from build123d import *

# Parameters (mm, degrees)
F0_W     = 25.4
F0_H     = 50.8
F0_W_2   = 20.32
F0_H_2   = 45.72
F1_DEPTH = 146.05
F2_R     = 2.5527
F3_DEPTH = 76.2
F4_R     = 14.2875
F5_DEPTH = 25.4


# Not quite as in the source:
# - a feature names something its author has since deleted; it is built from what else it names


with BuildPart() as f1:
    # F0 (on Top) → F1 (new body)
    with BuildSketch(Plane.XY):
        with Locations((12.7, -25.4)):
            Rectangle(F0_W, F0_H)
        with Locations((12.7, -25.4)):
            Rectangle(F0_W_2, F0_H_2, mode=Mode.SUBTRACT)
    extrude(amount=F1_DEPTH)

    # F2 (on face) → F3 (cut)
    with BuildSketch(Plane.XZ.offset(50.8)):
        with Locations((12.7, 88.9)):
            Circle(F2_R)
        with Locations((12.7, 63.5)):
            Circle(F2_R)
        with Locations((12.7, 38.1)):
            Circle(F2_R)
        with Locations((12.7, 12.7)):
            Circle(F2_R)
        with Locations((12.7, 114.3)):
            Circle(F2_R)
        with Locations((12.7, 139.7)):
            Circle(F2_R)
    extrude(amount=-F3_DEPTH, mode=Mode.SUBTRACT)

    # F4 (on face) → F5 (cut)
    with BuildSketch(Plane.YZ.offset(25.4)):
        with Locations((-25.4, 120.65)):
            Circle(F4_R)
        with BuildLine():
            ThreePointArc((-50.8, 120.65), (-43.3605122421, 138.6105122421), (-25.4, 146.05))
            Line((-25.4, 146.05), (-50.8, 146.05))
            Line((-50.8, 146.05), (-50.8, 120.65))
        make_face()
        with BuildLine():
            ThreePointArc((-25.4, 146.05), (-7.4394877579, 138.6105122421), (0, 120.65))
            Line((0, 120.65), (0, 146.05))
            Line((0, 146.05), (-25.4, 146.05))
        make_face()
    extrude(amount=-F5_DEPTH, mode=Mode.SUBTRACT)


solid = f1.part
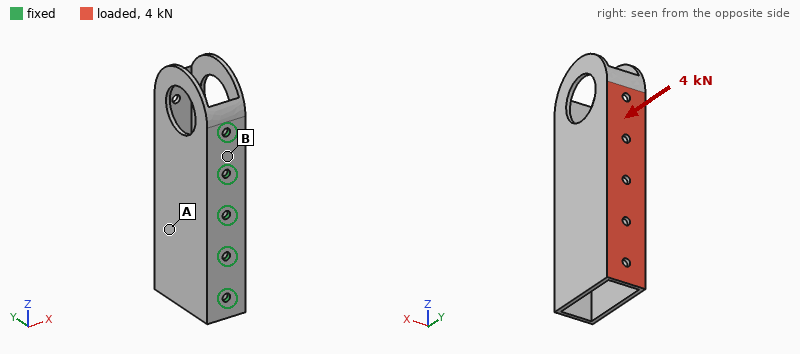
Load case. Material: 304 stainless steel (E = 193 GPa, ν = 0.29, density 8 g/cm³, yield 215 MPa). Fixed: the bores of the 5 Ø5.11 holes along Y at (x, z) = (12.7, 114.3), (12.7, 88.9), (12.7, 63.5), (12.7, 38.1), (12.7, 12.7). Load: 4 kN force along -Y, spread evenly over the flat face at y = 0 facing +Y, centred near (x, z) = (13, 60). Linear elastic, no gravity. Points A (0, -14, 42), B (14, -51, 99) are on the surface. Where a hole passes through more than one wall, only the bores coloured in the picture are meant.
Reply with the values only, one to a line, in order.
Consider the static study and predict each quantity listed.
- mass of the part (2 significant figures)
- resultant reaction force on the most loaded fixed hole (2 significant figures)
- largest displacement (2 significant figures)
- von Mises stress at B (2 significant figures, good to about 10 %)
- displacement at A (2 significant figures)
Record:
370 g
890 N
37 µm
65 MPa
25 µm
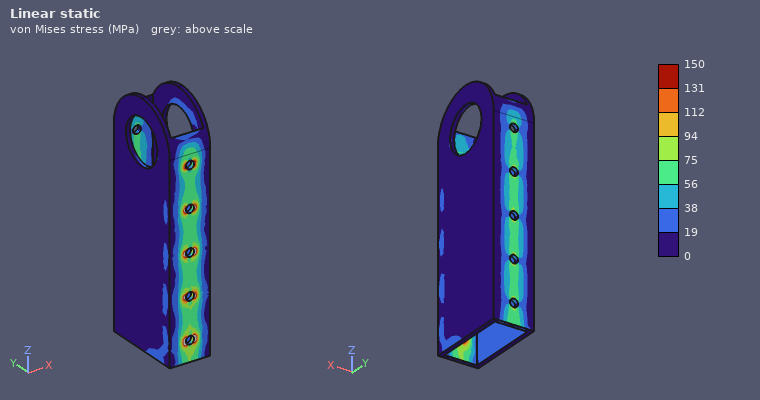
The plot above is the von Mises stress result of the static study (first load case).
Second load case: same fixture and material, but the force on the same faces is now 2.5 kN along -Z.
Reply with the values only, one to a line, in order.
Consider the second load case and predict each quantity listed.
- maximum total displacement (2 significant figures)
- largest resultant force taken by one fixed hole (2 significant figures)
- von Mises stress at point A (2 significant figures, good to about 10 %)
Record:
38 µm
1.1 kN
14 MPa
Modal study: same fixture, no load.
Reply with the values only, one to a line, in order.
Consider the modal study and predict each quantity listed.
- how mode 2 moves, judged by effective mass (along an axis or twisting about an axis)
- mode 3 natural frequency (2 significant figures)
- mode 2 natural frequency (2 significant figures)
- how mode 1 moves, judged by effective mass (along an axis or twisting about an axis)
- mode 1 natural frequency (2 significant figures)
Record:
twisting about Y
2700 Hz
1900 Hz
along X
670 Hz
